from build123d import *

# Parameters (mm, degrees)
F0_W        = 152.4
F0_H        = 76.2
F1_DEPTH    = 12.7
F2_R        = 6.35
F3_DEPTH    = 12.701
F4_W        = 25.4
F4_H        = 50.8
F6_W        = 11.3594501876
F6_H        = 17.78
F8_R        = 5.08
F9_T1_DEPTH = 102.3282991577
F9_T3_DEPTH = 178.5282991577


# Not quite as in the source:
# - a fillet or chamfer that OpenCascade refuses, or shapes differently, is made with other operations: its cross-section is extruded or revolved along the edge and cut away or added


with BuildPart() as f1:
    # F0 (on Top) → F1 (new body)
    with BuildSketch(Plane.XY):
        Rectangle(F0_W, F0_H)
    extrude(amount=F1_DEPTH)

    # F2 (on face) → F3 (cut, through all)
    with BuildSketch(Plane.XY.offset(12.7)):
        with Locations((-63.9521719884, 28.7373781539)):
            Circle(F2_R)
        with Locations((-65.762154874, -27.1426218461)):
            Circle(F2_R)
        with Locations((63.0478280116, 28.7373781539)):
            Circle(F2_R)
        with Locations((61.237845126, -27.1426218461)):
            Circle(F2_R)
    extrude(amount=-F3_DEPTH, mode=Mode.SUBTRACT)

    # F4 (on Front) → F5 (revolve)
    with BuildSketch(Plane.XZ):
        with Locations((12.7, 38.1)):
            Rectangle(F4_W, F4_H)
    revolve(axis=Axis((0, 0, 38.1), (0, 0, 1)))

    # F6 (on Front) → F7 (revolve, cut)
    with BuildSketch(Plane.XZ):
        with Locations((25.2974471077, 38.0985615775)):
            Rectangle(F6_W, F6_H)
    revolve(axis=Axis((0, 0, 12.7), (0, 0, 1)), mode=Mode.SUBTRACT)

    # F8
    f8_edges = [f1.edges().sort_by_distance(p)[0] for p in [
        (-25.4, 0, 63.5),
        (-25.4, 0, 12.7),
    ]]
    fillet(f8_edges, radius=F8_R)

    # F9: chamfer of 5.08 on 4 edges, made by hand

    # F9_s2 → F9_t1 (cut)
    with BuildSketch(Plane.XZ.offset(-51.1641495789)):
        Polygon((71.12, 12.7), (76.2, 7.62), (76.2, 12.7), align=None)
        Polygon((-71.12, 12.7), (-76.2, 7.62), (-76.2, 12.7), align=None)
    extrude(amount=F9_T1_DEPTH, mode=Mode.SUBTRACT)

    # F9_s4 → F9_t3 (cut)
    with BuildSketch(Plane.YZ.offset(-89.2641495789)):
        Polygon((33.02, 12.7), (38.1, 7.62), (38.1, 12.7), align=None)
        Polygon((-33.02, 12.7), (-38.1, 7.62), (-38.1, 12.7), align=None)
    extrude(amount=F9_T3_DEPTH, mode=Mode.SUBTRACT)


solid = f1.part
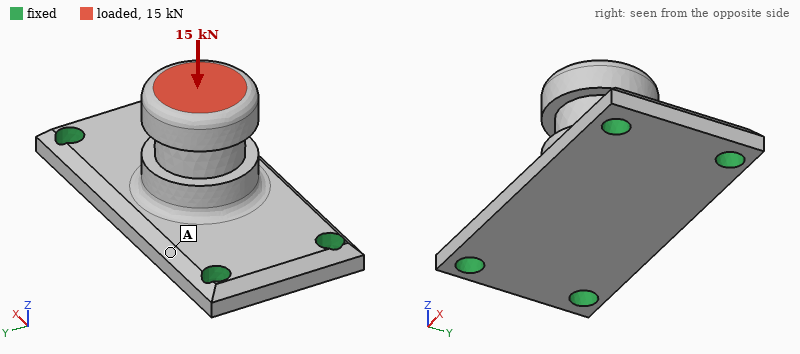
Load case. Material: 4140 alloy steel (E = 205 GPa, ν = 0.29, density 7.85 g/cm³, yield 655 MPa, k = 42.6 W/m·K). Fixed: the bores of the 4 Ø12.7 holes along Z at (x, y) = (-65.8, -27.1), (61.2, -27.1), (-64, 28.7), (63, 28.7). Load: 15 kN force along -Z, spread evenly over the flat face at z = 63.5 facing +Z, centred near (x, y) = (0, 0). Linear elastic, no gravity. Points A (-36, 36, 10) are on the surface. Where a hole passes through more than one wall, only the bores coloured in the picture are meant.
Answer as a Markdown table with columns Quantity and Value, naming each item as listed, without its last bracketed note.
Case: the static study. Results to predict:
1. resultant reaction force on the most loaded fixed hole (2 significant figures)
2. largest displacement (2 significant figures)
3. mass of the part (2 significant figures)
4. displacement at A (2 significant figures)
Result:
| Quantity | Value |
|---|---|
| resultant reaction force on the most loaded fixed hole | 4.5 kN |
| largest displacement | 34 µm |
| mass of the part | 1.8 kg |
| displacement at A | 16 µm |
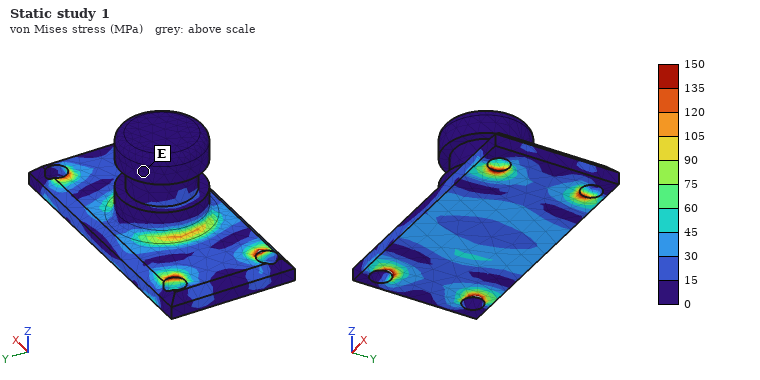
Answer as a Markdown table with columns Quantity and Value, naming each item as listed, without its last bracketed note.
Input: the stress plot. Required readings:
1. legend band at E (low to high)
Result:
| Quantity | Value |
|---|---|
| legend band at E | 0 to 15 MPa |
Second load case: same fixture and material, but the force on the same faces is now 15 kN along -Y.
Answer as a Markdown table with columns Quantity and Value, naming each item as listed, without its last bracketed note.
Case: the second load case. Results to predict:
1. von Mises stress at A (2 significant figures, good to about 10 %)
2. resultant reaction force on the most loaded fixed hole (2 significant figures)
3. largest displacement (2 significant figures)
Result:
| Quantity | Value |
|---|---|
| von Mises stress at A | 92 MPa |
| resultant reaction force on the most loaded fixed hole | 10 kN |
| largest displacement | 0.18 mm |
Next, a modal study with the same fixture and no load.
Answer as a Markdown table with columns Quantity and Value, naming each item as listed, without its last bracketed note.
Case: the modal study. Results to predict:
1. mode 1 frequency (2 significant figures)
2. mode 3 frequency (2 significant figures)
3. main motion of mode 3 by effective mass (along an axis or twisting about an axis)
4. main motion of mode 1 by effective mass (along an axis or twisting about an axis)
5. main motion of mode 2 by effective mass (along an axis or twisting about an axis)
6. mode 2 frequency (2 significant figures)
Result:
| Quantity | Value |
|---|---|
| mode 1 frequency | 2600 Hz |
| mode 3 frequency | 4200 Hz |
| main motion of mode 3 by effective mass | along X |
| main motion of mode 1 by effective mass | along Y |
| main motion of mode 2 by effective mass | along Z |
| mode 2 frequency | 3200 Hz |
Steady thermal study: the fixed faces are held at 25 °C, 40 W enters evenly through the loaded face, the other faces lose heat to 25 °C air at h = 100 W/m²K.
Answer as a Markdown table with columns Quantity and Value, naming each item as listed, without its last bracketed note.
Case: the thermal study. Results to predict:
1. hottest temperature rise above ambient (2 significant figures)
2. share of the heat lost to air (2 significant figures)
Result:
| Quantity | Value |
|---|---|
| hottest temperature rise above ambient | 34 K |
| share of the heat lost to air | 69 % |
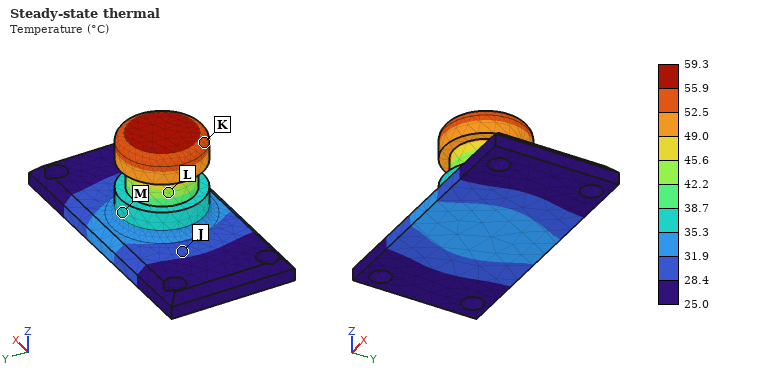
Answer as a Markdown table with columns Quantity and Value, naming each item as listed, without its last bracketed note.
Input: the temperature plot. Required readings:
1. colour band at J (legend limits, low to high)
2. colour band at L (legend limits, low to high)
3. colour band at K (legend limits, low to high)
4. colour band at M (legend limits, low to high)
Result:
| Quantity | Value |
|---|---|
| colour band at J | 28.4 to 31.9 °C |
| colour band at L | 42.2 to 45.6 °C |
| colour band at K | 52.5 to 55.9 °C |
| colour band at M | 35.3 to 38.7 °C |
